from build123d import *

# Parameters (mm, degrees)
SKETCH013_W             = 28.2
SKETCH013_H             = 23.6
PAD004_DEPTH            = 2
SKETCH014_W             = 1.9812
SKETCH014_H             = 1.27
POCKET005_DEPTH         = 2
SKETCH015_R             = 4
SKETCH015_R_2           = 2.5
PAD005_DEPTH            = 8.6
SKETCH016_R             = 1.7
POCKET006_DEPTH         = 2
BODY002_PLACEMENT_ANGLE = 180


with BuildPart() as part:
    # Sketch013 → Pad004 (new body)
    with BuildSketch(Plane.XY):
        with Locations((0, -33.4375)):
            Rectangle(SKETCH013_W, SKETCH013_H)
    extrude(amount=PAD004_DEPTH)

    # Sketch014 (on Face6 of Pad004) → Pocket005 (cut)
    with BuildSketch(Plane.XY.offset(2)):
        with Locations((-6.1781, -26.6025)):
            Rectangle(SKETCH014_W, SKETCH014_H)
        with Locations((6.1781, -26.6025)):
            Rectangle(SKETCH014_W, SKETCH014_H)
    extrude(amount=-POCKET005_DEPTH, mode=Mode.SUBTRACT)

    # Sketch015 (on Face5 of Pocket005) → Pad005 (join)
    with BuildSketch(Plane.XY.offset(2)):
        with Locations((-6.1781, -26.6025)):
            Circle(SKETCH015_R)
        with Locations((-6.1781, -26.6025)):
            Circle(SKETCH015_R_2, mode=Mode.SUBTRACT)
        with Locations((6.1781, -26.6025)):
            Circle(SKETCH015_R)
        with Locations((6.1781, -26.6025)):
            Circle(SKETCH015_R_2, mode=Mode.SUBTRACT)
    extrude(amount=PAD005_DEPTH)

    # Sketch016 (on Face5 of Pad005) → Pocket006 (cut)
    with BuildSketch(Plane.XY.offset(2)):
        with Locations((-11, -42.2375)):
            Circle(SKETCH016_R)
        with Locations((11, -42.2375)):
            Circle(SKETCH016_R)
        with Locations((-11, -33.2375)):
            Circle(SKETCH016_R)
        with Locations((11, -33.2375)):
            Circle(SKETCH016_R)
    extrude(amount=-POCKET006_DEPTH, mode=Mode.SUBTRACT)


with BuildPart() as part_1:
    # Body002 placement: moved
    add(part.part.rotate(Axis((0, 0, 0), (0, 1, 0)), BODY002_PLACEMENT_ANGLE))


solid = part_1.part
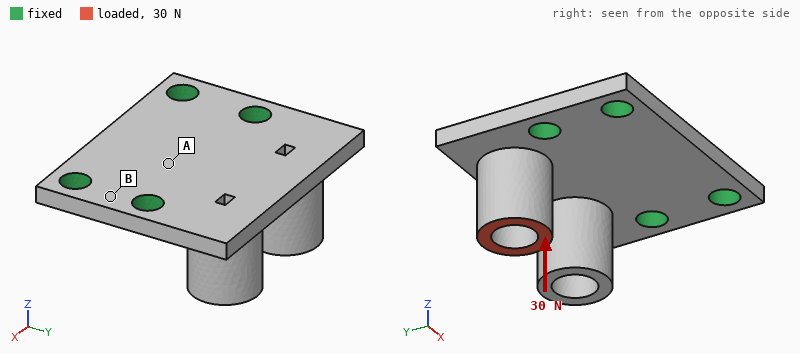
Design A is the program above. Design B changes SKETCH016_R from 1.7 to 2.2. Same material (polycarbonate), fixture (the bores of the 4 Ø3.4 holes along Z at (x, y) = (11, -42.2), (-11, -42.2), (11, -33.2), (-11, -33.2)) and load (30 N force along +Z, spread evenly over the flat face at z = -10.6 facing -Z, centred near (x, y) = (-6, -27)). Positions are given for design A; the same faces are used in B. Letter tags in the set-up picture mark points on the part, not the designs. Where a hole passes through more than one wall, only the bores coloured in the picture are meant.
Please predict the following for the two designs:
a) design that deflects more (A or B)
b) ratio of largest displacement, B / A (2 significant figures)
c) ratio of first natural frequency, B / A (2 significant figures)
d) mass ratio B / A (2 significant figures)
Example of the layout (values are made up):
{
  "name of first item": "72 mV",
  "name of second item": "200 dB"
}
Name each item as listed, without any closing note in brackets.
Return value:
{
  "design that deflects more": "A",
  "ratio of largest displacement, B / A": "0.84",
  "ratio of first natural frequency, B / A": "1.1",
  "mass ratio B / A": "0.97"
}
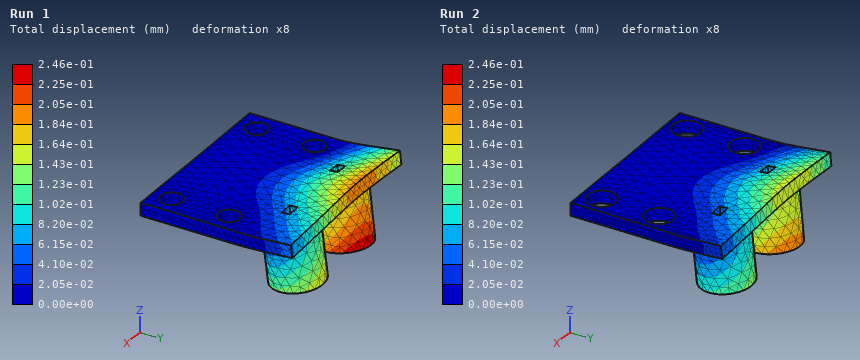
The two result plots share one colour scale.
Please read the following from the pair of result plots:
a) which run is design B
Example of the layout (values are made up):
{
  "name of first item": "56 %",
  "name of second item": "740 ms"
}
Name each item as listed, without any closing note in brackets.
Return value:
{
  "which run is design B": "Run 2"
}
